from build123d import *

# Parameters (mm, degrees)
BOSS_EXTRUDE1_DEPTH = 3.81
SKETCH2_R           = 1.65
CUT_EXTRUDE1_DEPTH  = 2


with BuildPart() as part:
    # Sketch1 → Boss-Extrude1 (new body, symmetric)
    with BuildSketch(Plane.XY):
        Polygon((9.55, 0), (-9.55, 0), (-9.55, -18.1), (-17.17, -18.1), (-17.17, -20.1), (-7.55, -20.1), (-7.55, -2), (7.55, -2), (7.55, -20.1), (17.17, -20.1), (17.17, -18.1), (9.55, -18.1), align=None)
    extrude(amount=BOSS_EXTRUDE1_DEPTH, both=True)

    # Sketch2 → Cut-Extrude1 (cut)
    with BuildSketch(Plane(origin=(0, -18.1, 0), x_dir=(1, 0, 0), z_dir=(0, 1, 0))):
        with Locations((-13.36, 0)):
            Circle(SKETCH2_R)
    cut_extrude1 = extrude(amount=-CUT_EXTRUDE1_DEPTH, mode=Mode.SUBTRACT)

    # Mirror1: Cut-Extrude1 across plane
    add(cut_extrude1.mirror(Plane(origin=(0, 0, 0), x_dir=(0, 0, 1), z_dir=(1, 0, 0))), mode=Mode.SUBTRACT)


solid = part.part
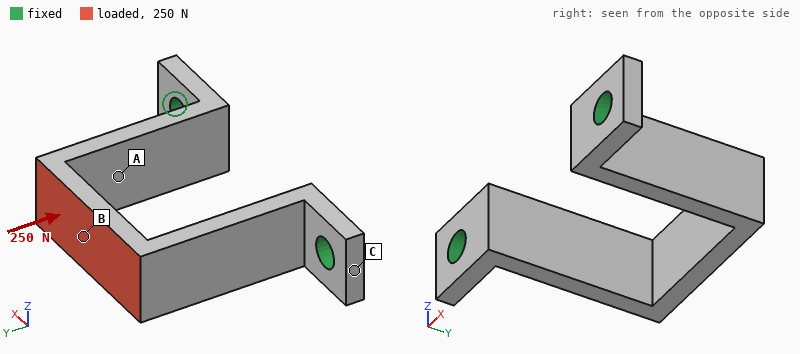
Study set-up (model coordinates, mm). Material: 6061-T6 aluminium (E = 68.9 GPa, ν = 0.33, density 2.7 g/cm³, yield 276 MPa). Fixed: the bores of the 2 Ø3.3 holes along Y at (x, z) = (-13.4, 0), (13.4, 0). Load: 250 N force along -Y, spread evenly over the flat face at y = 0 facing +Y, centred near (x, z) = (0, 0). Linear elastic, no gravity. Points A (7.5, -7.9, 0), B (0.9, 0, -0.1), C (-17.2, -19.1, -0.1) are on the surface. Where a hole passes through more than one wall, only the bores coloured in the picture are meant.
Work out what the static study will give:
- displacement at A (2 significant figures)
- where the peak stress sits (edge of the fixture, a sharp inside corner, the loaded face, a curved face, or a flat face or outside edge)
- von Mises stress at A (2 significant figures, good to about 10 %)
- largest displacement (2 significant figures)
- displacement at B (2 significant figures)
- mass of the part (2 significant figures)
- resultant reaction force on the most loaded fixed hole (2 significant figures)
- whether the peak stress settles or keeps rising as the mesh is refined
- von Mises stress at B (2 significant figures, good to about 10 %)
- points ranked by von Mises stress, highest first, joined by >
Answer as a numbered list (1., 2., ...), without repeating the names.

1. 6.5 µm
2. edge of the fixture
3. 23 MPa
4. 24 µm
5. 22 µm
6. 2.8 g
7. 130 N
8. keeps rising
9. 44 MPa
10. B > A > C
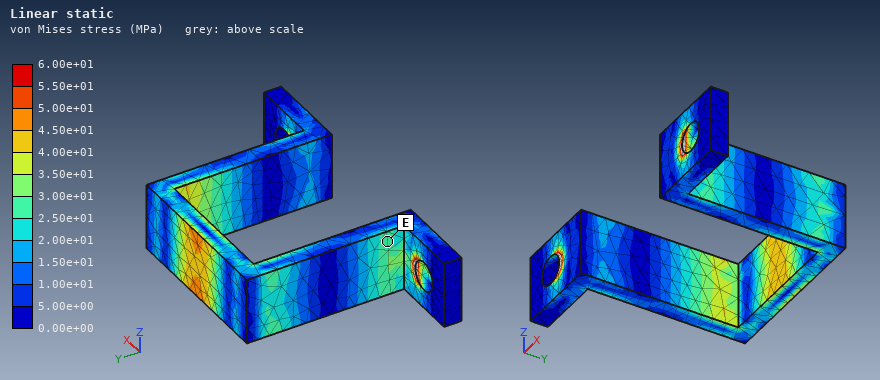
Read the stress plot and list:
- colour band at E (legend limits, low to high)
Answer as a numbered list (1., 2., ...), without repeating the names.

1. 2.50e+01 to 3.00e+01 MPa
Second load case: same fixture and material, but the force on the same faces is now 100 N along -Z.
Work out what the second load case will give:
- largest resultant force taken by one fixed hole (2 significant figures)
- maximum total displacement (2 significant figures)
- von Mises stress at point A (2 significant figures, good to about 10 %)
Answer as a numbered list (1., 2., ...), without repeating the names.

1. 50 N
2. 0.12 mm
3. 18 MPa
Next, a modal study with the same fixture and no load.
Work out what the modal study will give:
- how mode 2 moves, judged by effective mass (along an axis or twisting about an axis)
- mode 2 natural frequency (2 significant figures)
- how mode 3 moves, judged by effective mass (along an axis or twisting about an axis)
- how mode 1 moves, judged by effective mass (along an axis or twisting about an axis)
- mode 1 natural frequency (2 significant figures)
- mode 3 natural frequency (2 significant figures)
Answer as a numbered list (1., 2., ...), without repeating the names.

1. along Z
2. 4500 Hz
3. twisting about Y
4. along X
5. 4200 Hz
6. 7700 Hz
